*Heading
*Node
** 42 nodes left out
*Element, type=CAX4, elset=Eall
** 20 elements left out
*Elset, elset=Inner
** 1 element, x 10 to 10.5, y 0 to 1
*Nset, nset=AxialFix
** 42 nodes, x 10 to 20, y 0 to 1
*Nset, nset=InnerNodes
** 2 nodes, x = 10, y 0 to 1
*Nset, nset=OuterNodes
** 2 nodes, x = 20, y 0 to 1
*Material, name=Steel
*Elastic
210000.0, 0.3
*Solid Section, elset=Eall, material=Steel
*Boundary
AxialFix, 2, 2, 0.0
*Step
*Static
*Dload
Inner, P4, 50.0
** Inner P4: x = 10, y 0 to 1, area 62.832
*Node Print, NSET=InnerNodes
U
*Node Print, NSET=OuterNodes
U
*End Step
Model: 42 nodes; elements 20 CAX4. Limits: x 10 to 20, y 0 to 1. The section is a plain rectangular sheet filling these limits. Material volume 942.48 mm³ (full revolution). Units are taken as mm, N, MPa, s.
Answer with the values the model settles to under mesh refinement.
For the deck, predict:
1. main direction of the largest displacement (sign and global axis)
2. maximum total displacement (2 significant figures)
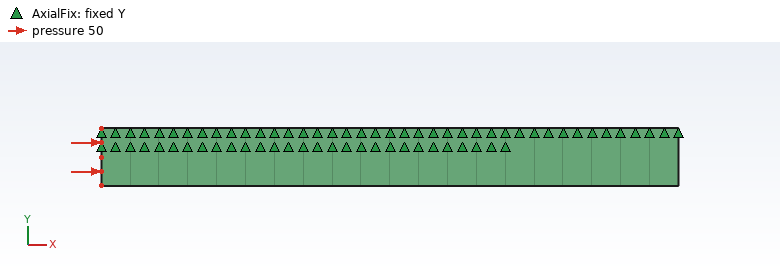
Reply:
+X
0.0045 mm
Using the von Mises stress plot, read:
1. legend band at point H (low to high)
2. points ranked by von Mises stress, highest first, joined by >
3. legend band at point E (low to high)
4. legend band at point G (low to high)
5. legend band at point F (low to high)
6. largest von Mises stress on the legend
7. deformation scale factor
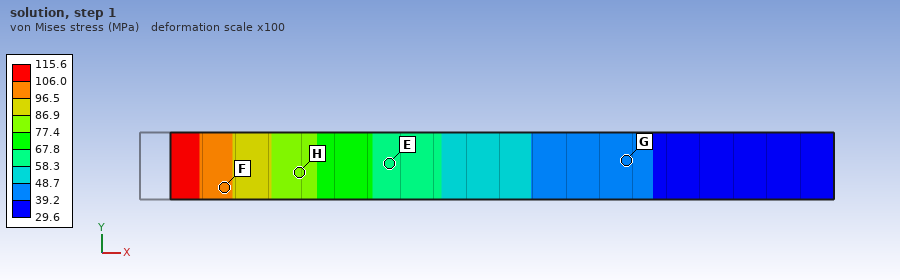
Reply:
77.4 to 86.9 MPa
F > H > E > G
58.3 to 67.8 MPa
39.2 to 48.7 MPa
96.5 to 106.0 MPa
115.6 MPa
100
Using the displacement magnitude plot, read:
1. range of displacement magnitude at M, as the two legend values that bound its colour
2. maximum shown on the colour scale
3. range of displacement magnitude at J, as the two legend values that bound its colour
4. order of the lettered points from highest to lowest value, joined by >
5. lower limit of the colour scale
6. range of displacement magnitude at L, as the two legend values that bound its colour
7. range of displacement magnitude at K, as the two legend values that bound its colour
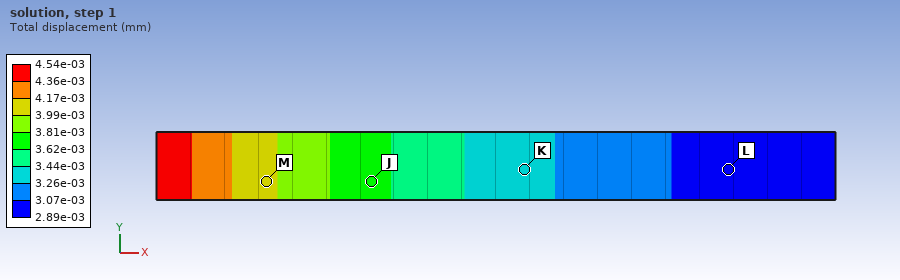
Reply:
3.99e-03 to 4.17e-03 mm
4.54e-03 mm
3.62e-03 to 3.81e-03 mm
M > J > K > L
2.89e-03 mm
2.89e-03 to 3.07e-03 mm
3.26e-03 to 3.44e-03 mm
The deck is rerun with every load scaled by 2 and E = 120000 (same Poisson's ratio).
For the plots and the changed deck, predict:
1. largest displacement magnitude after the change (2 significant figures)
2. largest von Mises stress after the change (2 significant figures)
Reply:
0.016 mm
230 MPa
